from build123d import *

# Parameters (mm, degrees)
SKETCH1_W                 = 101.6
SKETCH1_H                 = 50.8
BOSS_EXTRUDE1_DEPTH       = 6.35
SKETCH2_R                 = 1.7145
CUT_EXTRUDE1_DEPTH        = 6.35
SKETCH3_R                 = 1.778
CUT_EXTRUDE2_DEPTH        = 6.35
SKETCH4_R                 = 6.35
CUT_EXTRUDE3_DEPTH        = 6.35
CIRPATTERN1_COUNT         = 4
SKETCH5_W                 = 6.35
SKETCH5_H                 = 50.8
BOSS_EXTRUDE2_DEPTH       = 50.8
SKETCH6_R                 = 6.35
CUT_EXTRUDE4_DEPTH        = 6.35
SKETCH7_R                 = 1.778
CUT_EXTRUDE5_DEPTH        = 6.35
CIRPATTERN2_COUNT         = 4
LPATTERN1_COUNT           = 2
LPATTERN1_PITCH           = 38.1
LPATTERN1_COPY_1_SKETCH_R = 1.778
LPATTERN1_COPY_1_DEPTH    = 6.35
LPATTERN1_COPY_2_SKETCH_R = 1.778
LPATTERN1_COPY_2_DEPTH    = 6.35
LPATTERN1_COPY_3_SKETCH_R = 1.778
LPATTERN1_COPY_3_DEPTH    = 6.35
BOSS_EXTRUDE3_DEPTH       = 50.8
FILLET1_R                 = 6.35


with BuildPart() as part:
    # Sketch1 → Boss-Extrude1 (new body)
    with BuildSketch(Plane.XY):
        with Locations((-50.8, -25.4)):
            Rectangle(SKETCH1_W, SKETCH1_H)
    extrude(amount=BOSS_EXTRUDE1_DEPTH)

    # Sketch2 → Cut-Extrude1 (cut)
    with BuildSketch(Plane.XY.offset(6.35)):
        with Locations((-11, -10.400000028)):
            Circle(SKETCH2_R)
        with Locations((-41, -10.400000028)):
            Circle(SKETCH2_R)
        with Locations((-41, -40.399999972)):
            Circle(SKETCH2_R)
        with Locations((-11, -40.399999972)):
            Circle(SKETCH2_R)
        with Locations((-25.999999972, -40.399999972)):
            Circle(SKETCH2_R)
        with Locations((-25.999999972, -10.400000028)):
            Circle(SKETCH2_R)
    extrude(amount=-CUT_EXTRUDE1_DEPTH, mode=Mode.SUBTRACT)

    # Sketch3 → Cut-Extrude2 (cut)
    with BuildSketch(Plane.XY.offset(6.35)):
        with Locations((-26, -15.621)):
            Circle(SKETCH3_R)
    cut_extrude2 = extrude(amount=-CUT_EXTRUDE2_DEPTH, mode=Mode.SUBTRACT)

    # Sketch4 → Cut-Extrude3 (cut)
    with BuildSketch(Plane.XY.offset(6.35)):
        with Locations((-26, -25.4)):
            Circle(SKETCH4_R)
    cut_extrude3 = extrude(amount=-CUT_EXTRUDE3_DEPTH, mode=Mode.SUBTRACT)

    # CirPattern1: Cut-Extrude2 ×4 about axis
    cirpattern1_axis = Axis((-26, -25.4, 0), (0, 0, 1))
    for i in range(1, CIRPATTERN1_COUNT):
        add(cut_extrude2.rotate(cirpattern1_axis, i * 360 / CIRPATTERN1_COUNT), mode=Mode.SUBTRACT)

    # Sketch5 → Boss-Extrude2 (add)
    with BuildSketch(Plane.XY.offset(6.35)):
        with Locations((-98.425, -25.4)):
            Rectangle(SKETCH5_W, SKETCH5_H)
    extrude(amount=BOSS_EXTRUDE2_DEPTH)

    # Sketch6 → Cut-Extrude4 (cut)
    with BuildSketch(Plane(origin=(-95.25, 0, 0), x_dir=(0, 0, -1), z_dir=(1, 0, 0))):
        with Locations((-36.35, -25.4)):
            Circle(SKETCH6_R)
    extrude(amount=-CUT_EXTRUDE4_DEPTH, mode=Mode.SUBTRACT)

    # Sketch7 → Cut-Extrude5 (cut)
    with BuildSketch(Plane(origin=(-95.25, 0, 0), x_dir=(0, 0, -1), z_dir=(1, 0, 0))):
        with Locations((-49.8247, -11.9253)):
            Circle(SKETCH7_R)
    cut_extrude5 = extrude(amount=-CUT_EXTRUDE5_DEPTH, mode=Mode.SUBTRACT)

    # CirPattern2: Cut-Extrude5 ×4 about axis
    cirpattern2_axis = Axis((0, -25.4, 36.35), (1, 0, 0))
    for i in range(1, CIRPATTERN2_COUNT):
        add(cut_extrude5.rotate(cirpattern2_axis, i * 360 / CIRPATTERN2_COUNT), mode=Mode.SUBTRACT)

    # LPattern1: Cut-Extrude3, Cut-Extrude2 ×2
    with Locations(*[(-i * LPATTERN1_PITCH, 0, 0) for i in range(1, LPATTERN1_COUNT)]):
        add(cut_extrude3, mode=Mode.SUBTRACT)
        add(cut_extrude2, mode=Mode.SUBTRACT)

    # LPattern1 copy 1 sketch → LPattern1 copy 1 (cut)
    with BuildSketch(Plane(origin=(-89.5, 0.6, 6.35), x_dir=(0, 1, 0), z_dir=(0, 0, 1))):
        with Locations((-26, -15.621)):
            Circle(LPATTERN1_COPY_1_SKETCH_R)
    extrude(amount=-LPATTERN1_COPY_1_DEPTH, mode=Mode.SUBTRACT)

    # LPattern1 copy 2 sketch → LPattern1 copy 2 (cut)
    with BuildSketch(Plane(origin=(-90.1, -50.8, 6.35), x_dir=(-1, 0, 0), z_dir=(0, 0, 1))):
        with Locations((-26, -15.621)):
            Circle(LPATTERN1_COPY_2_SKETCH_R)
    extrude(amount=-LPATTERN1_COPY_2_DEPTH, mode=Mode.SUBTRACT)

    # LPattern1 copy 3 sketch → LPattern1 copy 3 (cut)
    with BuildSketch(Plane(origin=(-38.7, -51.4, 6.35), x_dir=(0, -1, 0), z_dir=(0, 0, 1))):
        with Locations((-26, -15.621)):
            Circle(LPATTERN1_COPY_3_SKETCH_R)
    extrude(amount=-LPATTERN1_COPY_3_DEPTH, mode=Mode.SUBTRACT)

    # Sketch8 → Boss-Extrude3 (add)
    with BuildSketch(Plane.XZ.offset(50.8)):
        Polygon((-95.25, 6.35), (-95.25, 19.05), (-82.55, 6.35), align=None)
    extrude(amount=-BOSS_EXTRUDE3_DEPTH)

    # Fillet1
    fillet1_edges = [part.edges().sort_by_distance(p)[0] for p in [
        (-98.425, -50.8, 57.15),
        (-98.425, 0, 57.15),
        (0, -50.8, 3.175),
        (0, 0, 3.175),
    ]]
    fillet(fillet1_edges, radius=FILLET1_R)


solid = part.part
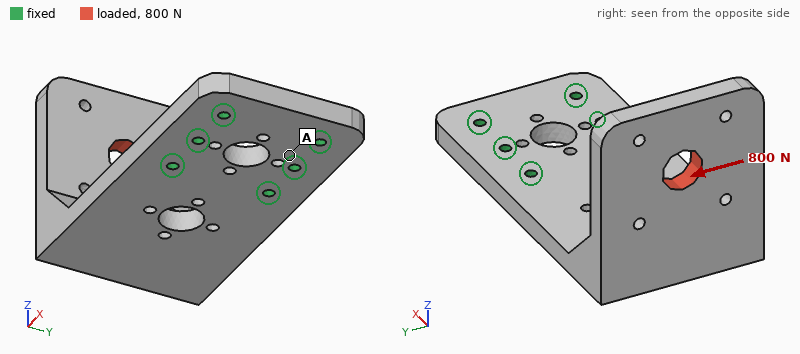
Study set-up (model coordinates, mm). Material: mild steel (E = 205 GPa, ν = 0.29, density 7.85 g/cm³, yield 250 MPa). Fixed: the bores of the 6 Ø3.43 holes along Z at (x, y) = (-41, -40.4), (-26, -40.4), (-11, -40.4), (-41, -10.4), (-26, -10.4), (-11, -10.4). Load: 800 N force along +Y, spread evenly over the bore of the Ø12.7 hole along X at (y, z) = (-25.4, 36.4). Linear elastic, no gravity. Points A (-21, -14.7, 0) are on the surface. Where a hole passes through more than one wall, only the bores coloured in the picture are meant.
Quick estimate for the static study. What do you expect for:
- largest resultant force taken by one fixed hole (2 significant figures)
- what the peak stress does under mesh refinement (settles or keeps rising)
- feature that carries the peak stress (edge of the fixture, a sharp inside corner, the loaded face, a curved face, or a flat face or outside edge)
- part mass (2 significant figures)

1.4 kN
keeps rising
edge of the fixture
390 g
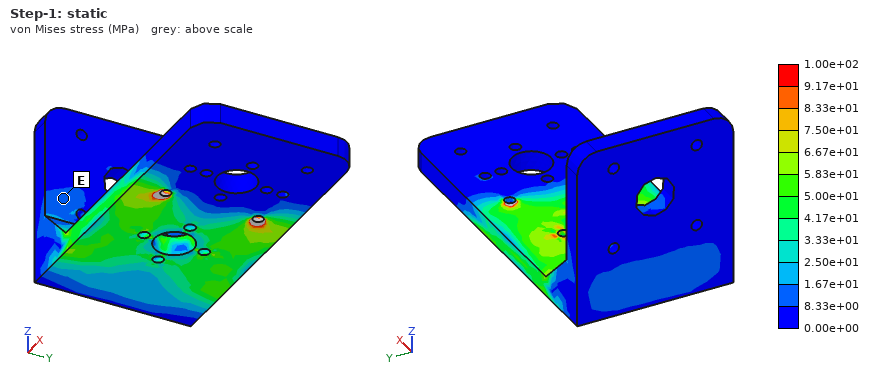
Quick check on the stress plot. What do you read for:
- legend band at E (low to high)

8.33e+00 to 1.67e+01 MPa
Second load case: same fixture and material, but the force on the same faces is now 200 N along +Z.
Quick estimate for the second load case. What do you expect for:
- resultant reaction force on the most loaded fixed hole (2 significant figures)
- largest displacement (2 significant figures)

260 N
0.12 mm
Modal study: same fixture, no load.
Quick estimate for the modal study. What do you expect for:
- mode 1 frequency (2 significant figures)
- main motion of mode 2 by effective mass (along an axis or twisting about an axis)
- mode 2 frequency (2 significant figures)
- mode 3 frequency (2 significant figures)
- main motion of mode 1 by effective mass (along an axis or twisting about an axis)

530 Hz
along Y
1200 Hz
2200 Hz
along Z
